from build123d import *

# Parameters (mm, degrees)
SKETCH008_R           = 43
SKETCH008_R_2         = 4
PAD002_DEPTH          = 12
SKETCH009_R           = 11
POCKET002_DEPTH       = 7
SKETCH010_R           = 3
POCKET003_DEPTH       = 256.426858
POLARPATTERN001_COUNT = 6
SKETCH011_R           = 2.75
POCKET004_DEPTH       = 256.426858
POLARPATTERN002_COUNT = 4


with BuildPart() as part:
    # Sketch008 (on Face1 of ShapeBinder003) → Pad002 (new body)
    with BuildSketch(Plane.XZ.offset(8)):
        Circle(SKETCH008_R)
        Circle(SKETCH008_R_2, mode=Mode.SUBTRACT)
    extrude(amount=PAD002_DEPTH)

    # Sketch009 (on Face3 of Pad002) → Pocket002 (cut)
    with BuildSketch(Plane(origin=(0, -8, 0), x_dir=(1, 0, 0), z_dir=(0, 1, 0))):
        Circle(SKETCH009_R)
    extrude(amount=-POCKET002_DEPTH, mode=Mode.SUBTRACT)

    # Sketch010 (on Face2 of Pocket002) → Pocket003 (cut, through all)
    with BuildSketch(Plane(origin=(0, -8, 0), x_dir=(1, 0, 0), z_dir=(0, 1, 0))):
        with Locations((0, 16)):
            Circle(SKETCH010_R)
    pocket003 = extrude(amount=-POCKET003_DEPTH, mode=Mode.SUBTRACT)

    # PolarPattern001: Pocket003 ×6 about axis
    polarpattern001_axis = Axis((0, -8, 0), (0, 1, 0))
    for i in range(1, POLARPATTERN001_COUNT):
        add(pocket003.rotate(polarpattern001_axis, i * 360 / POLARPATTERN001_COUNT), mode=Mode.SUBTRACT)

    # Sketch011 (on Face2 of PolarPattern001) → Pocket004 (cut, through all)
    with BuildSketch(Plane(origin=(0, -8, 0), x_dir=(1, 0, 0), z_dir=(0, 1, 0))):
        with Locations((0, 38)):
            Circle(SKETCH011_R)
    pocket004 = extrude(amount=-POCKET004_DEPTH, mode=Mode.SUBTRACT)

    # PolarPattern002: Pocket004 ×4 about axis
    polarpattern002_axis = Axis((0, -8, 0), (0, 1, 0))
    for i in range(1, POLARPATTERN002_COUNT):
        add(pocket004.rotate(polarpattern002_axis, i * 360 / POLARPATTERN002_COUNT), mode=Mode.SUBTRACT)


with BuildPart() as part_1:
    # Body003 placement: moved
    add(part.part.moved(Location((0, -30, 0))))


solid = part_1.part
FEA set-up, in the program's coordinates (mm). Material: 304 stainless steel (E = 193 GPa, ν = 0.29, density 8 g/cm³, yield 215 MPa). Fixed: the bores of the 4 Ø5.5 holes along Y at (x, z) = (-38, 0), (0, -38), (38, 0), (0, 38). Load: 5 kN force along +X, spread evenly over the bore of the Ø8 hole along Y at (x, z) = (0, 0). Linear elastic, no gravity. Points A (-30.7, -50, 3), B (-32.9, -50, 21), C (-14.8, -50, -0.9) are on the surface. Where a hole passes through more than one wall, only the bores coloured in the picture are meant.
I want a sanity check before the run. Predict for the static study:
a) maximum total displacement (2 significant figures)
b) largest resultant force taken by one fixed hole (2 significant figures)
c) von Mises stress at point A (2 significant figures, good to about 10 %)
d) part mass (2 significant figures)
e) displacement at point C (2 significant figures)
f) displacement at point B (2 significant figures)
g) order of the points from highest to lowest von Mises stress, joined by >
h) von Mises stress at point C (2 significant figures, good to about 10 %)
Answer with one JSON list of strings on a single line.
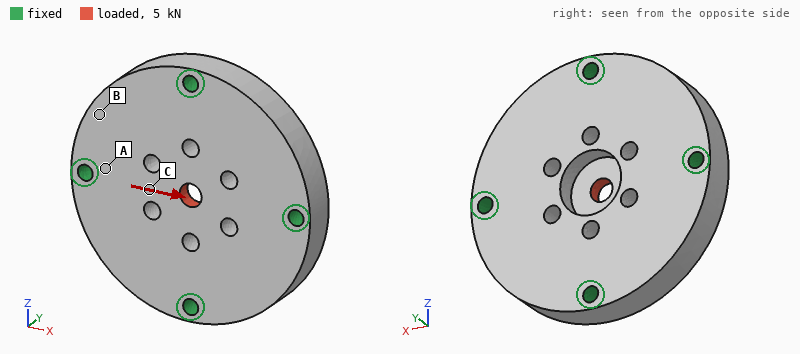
["3.2 µm", "1.7 kN", "11 MPa", "510 g", "1.5 µm", "0.70 µm", "C > A > B", "19 MPa"]
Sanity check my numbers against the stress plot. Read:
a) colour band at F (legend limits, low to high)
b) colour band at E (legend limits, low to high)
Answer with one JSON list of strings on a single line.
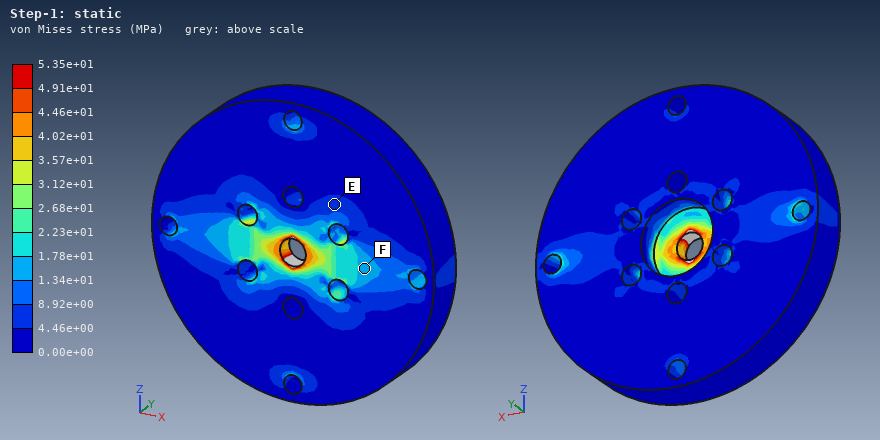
["1.34e+01 to 1.78e+01 MPa", "4.46e+00 to 8.92e+00 MPa"]
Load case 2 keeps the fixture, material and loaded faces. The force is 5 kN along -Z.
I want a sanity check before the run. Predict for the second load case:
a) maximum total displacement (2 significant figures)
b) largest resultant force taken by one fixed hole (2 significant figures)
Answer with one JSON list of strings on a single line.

["3.3 µm", "1.6 kN"]
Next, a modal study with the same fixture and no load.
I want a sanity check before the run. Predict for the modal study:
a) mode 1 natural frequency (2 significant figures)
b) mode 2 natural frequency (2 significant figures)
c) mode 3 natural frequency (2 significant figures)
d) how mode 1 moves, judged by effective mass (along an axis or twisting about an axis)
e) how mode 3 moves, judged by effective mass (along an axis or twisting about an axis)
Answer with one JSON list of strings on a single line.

["12 kHz", "14 kHz", "14 kHz", "along Y", "twisting about Z"]
